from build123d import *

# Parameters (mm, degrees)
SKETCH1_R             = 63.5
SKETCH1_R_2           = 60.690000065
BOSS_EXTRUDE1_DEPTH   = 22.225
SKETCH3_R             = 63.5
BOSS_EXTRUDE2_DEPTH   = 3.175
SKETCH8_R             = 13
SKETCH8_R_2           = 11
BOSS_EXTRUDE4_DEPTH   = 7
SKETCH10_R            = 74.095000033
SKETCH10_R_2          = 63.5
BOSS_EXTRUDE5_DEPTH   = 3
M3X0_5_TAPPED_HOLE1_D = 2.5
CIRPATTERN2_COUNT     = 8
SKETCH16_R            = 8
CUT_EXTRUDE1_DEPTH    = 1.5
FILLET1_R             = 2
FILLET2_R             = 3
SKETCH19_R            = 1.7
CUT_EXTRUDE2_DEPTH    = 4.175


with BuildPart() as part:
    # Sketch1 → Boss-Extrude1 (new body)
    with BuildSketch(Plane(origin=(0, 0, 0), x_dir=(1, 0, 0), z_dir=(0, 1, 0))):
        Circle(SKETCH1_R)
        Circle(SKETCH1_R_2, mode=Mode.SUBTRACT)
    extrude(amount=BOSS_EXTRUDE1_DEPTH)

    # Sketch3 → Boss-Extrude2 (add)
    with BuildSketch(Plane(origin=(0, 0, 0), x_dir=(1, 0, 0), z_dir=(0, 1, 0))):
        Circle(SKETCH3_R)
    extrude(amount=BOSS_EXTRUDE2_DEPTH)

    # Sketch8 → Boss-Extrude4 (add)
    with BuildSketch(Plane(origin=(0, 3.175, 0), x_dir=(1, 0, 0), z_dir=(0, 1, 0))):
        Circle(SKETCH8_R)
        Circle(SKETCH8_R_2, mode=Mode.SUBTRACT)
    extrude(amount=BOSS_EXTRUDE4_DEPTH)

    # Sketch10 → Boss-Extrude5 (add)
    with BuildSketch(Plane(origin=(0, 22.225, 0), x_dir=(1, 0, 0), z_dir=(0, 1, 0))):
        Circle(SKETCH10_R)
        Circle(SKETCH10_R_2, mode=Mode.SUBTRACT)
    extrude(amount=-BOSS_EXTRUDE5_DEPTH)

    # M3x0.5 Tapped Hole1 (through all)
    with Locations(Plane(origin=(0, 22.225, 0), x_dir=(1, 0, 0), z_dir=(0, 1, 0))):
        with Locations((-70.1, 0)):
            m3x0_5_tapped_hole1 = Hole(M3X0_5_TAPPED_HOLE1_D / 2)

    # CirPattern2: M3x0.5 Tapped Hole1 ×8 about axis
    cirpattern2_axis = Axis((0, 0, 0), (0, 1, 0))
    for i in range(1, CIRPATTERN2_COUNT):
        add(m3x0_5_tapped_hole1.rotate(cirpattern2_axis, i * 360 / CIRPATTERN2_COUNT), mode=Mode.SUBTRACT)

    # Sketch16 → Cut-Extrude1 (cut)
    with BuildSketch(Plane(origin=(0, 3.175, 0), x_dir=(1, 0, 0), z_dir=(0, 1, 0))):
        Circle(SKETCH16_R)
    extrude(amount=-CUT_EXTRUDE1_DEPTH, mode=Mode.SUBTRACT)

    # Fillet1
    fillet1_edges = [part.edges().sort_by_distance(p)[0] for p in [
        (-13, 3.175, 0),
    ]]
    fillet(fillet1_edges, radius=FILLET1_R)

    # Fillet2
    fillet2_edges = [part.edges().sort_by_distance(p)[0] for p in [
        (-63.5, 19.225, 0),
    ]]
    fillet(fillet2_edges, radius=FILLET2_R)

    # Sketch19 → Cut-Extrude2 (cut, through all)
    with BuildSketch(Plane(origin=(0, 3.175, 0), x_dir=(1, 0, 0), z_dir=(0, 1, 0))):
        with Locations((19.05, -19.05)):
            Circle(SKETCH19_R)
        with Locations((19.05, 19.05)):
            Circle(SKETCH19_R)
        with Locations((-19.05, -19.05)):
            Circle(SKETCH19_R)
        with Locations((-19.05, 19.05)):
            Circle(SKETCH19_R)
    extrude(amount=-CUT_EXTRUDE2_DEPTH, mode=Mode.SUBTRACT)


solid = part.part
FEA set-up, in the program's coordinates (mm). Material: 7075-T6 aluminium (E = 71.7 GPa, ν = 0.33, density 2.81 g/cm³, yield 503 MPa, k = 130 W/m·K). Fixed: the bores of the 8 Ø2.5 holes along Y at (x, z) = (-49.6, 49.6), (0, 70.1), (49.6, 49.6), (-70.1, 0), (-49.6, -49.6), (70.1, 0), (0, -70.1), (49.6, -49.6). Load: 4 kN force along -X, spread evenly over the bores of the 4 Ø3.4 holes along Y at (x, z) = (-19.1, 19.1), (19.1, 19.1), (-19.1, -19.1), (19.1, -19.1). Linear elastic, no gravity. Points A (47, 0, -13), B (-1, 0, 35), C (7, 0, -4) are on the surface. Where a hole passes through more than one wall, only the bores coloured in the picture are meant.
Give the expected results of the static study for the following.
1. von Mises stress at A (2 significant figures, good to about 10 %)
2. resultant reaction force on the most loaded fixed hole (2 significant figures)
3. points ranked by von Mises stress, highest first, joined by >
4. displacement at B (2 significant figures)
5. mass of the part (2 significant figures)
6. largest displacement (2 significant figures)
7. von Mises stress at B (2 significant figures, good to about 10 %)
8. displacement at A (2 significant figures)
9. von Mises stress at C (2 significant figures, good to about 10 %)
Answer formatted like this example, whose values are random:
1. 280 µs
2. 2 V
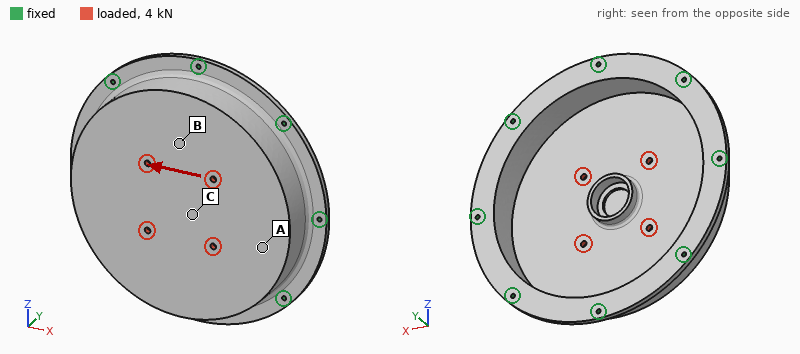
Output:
1. 11 MPa
2. 740 N
3. A > B > C
4. 17 µm
5. 210 g
6. 26 µm
7. 8.2 MPa
8. 21 µm
9. 3.5 MPa
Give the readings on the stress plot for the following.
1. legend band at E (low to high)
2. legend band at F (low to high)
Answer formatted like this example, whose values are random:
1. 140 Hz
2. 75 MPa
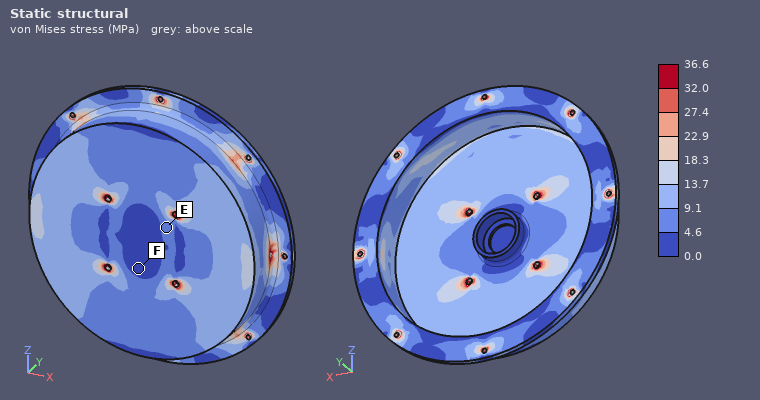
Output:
1. 4.6 to 9.1 MPa
2. 0.0 to 4.6 MPa
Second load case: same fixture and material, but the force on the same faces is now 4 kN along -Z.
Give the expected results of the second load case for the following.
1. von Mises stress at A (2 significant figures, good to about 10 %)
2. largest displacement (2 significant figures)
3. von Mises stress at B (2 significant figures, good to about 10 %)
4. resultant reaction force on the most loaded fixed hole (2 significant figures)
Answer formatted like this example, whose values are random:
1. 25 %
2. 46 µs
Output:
1. 6.5 MPa
2. 26 µm
3. 7.3 MPa
4. 740 N
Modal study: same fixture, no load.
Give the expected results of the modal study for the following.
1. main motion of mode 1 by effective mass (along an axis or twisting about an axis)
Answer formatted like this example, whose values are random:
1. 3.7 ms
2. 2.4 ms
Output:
1. along Y
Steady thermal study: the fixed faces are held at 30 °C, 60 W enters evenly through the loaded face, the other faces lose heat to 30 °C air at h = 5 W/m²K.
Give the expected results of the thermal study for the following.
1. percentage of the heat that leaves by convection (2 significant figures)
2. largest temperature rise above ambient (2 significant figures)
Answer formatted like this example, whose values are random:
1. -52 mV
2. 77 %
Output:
1. 7.4 %
2. 43 K
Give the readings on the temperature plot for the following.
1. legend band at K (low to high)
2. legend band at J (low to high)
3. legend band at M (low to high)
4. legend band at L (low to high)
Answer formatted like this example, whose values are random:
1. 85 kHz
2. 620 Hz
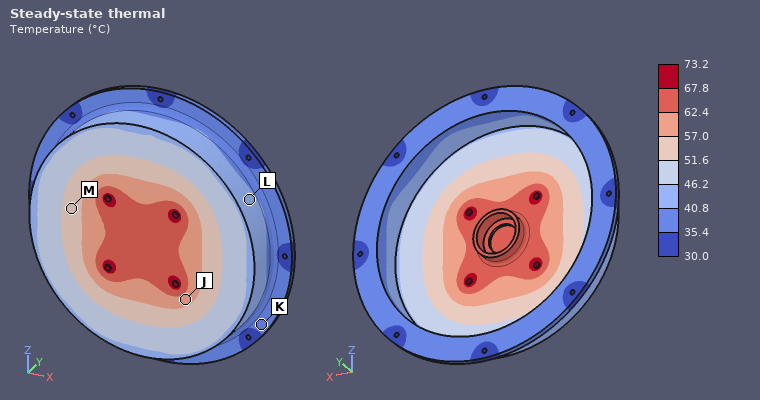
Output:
1. 35.4 to 40.8 °C
2. 57.0 to 62.4 °C
3. 51.6 to 57.0 °C
4. 40.8 to 46.2 °C
